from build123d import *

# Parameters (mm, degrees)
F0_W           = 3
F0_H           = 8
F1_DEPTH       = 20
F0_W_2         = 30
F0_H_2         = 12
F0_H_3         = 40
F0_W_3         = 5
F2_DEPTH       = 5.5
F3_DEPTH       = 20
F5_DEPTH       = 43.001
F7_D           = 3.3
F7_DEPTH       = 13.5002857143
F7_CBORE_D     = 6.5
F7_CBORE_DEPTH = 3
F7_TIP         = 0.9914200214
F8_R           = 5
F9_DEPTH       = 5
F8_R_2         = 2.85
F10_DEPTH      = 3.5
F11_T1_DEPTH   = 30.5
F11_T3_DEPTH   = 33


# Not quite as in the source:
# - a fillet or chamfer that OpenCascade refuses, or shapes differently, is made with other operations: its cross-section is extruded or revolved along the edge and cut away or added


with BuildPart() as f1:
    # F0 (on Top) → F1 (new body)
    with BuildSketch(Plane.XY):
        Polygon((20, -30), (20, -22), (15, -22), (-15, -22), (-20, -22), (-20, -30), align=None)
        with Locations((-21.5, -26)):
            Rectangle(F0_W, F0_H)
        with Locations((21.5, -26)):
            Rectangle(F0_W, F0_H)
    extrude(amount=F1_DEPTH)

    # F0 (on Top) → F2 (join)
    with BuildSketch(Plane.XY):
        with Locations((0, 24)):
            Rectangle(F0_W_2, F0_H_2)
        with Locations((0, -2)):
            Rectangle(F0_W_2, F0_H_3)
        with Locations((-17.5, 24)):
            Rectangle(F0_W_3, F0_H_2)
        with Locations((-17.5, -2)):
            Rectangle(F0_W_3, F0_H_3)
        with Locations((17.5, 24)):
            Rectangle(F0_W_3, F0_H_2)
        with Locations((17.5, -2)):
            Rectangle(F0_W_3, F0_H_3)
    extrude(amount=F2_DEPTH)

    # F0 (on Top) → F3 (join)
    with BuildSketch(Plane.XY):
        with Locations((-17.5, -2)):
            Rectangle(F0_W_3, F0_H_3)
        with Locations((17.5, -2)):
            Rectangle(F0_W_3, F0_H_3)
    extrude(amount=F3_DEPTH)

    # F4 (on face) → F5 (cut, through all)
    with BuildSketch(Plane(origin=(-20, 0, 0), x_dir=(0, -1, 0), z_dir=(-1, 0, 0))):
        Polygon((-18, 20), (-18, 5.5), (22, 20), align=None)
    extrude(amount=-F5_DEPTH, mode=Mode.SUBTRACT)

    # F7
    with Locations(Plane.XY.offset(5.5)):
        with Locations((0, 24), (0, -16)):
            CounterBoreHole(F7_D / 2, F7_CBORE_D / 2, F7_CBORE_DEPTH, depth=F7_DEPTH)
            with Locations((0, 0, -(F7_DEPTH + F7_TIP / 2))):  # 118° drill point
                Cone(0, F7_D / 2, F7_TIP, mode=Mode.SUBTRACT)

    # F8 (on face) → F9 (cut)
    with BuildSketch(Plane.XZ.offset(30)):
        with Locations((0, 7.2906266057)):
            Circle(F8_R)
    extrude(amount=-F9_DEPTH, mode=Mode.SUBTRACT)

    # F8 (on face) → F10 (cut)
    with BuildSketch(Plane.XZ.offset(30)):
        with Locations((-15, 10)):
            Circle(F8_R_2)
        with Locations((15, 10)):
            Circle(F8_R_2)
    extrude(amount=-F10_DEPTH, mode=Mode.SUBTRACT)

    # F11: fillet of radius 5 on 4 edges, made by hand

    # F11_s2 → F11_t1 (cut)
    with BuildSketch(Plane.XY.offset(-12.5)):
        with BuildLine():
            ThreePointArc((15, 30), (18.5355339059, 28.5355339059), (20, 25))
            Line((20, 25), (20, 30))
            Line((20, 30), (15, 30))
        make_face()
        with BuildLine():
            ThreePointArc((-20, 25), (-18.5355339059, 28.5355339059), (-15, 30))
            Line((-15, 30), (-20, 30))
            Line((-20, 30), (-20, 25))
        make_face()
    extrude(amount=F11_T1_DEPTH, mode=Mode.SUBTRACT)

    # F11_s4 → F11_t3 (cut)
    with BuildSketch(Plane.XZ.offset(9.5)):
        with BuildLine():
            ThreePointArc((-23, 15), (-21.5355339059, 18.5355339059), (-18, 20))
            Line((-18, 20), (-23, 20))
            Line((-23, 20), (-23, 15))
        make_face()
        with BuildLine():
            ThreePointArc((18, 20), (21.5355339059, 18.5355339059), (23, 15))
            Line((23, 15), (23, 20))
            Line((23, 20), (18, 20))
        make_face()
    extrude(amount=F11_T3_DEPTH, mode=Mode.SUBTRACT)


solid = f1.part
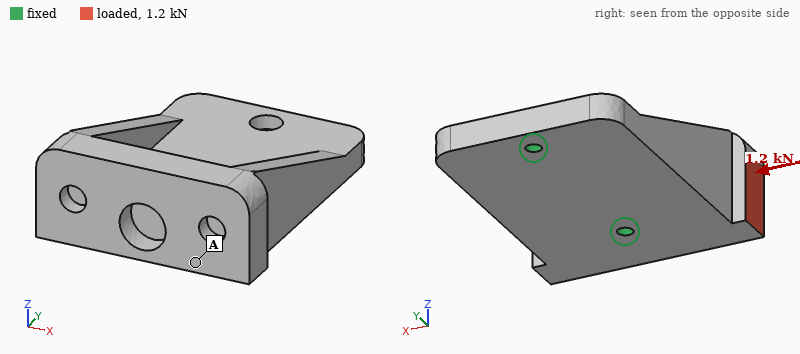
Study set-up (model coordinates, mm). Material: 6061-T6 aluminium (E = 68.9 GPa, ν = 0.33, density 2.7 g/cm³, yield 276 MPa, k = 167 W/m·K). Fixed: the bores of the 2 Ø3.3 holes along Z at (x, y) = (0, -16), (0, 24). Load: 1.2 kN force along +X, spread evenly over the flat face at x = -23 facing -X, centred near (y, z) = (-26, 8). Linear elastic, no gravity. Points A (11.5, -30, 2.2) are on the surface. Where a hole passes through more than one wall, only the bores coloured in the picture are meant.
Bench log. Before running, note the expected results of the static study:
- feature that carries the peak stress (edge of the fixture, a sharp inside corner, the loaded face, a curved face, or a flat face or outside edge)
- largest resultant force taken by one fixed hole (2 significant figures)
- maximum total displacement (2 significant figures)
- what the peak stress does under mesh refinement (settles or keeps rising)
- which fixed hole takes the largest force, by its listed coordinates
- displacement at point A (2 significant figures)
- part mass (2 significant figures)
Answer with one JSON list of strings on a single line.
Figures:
["edge of the fixture", "1.5 kN", "0.12 mm", "keeps rising", "(0, -16)", "0.049 mm", "56 g"]
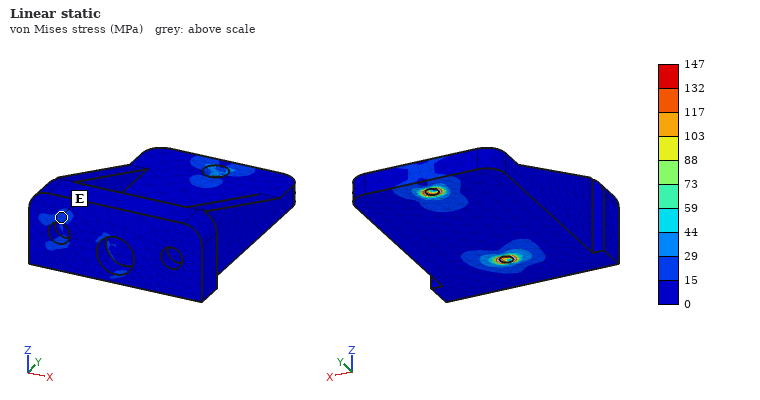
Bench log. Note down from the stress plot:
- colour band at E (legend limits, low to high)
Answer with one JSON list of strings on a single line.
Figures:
["15 to 29 MPa"]
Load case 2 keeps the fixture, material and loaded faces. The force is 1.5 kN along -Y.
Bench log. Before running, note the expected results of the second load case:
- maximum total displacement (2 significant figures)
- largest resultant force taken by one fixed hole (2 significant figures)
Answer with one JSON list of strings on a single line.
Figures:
["38 µm", "1.2 kN"]
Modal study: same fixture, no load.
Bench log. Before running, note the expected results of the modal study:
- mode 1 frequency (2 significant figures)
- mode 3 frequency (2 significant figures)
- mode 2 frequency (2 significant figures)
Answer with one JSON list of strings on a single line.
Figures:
["2100 Hz", "7300 Hz", "6200 Hz"]
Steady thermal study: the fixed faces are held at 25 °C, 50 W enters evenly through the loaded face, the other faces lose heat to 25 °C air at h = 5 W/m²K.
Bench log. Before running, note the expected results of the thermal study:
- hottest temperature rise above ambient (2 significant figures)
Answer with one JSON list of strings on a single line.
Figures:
["56 K"]
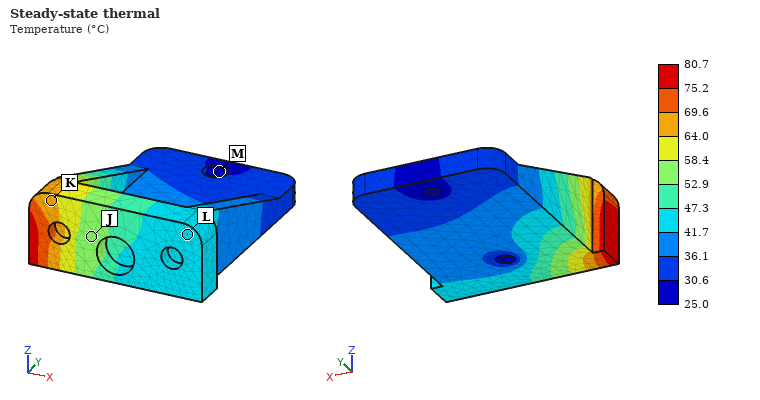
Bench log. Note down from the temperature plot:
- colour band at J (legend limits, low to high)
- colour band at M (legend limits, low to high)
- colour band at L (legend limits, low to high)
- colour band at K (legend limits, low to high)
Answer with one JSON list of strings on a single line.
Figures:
["52.9 to 58.4 °C", "25.0 to 30.6 °C", "41.7 to 47.3 °C", "64.0 to 69.6 °C"]
